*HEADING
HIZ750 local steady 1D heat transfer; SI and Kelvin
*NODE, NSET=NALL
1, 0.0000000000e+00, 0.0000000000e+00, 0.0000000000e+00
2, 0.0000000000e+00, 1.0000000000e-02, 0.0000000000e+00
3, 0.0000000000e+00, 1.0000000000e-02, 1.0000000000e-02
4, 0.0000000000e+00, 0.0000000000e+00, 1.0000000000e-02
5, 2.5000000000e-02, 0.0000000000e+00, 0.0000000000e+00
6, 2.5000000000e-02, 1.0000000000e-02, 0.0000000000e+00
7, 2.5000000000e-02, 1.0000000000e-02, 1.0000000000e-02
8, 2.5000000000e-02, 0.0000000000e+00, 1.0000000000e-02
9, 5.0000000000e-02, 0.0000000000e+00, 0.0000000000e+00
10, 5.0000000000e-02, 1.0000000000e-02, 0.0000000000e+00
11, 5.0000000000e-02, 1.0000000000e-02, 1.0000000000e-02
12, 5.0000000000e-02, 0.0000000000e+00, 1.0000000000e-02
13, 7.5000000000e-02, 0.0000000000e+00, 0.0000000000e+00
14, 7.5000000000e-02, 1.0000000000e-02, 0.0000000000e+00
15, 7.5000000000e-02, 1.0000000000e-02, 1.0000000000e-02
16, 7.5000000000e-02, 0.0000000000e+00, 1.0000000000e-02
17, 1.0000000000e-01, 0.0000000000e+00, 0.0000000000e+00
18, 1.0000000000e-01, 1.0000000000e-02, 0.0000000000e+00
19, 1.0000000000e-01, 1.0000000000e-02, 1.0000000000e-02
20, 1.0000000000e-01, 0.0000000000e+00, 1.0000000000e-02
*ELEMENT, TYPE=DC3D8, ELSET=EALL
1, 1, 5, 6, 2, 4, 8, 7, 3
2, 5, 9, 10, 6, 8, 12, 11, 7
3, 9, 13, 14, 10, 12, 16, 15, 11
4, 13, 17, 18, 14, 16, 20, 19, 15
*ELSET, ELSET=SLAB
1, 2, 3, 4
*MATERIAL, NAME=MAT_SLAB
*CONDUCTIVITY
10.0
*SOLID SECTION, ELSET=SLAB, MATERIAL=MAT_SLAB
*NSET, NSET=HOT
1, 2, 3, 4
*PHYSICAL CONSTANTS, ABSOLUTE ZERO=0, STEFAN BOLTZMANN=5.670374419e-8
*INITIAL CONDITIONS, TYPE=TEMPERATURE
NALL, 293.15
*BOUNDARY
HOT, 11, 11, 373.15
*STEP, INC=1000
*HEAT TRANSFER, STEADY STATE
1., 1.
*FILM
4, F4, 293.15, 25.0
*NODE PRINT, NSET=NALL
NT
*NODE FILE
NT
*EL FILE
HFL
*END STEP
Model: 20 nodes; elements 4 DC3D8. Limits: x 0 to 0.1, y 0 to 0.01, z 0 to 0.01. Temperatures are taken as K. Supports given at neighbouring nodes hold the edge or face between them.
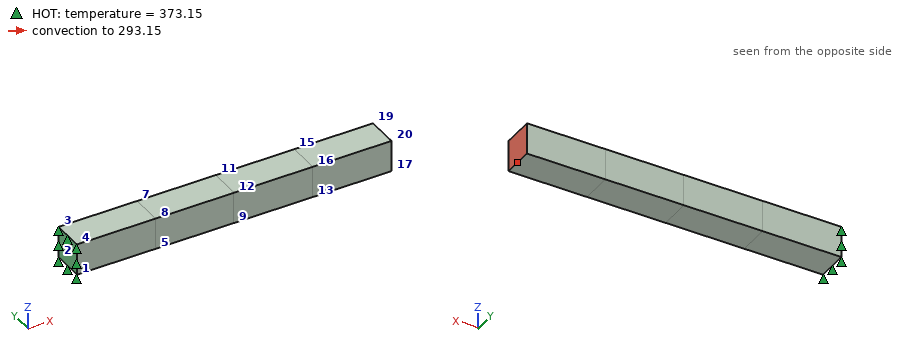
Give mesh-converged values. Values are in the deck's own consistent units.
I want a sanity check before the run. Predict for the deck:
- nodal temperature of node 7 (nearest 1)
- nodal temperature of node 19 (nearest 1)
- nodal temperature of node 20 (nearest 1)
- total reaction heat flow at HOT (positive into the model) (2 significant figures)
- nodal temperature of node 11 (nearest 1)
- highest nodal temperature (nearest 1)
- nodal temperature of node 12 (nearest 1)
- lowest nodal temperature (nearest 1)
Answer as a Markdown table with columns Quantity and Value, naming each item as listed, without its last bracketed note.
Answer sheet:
| Quantity | Value |
|---|---|
| nodal temperature of node 7 | 369 K |
| nodal temperature of node 19 | 357 K |
| nodal temperature of node 20 | 357 K |
| total reaction heat flow at HOT (positive into the model) | 0.16 |
| nodal temperature of node 11 | 365 K |
| highest nodal temperature | 373 K |
| nodal temperature of node 12 | 365 K |
| lowest nodal temperature | 357 K |
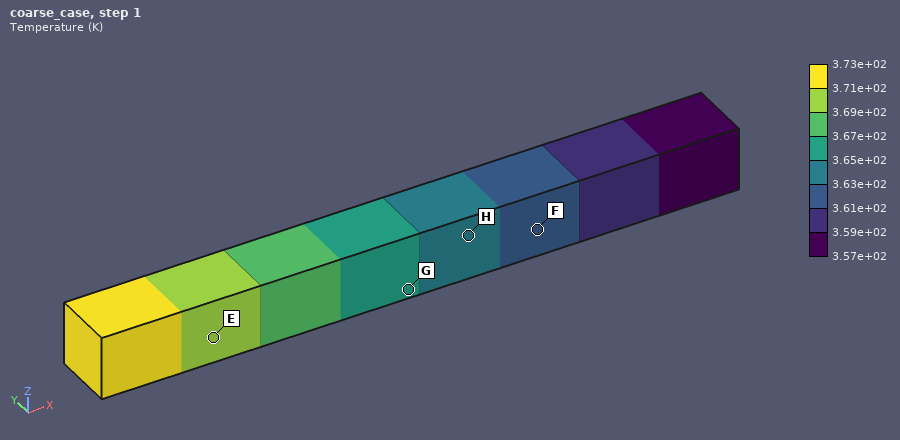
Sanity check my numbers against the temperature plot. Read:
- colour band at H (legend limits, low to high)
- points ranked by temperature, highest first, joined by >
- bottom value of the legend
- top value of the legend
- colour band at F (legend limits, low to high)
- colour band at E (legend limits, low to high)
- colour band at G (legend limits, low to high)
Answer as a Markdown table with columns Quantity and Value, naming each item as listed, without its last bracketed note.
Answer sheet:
| Quantity | Value |
|---|---|
| colour band at H | 3.63e+02 to 3.65e+02 K |
| points ranked by temperature, highest first, joined by > | E > G > H > F |
| bottom value of the legend | 3.57e+02 K |
| top value of the legend | 3.73e+02 K |
| colour band at F | 3.61e+02 to 3.63e+02 K |
| colour band at E | 3.69e+02 to 3.71e+02 K |
| colour band at G | 3.65e+02 to 3.67e+02 K |
